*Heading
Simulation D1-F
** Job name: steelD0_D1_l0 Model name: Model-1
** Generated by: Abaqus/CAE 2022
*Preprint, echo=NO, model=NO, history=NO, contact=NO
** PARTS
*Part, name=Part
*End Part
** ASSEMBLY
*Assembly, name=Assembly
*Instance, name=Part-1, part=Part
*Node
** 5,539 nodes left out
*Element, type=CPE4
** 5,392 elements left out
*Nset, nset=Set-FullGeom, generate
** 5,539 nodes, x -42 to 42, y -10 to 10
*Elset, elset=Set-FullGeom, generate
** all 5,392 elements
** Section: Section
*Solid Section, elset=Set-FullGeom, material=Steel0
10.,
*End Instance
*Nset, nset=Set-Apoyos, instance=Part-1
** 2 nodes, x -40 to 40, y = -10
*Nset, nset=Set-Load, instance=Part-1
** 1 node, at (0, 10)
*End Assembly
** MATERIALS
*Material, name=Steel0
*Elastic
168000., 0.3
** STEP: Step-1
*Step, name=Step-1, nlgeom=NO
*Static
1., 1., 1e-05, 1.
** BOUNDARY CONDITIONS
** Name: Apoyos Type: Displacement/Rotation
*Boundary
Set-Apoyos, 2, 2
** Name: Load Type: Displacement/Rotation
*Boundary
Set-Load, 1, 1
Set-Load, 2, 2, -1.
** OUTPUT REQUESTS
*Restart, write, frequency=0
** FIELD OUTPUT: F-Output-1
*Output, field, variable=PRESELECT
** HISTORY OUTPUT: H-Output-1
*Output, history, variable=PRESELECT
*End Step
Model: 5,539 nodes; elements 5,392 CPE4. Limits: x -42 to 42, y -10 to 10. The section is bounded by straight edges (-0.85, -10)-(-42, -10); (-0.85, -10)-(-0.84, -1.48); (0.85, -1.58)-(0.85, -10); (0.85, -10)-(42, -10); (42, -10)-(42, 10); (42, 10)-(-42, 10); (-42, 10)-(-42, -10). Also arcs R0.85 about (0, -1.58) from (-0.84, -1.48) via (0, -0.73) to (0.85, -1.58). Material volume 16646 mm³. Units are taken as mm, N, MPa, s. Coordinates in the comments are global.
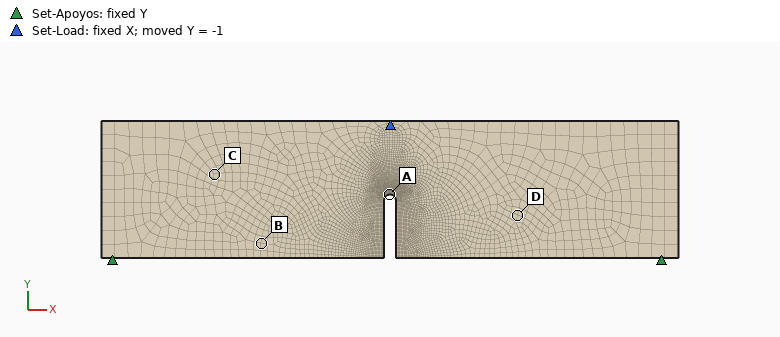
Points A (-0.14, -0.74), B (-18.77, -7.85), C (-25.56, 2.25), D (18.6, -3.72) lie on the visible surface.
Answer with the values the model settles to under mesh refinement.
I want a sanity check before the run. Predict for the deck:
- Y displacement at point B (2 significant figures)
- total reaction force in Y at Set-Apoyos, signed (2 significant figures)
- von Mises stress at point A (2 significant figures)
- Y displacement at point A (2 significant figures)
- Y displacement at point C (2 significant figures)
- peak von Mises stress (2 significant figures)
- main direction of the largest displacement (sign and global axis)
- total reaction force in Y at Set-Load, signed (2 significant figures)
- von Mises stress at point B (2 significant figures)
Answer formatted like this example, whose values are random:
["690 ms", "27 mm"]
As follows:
["-0.59 mm", "34000 N", "8700 MPa", "-0.98 mm", "-0.42 mm", "9100 MPa", "-Y", "-34000 N", "370 MPa"]
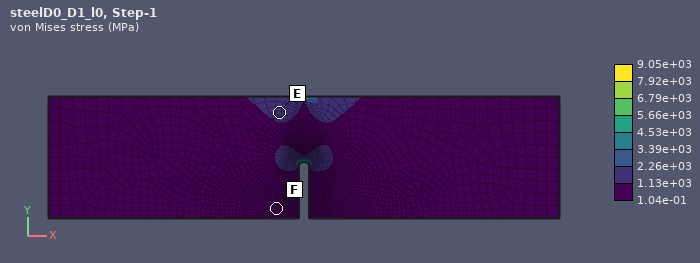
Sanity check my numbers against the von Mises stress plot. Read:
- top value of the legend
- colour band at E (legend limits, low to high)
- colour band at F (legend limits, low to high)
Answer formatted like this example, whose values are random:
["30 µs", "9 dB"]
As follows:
["9.05e+03 MPa", "1.13e+03 to 2.26e+03 MPa", "1.04e-01 to 1.13e+03 MPa"]
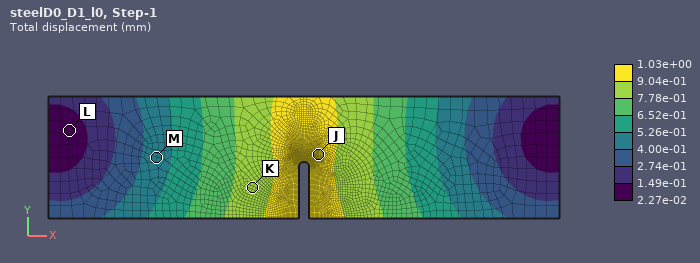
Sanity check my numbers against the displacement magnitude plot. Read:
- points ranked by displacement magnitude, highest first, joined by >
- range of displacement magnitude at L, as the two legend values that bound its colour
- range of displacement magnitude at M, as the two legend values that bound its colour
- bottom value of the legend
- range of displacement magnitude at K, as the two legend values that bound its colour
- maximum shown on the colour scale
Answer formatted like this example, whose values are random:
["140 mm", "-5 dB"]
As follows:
["J > K > M > L", "2.27e-02 to 1.49e-01 mm", "4.00e-01 to 5.26e-01 mm", "2.27e-02 mm", "7.78e-01 to 9.04e-01 mm", "1.03e+00 mm"]
